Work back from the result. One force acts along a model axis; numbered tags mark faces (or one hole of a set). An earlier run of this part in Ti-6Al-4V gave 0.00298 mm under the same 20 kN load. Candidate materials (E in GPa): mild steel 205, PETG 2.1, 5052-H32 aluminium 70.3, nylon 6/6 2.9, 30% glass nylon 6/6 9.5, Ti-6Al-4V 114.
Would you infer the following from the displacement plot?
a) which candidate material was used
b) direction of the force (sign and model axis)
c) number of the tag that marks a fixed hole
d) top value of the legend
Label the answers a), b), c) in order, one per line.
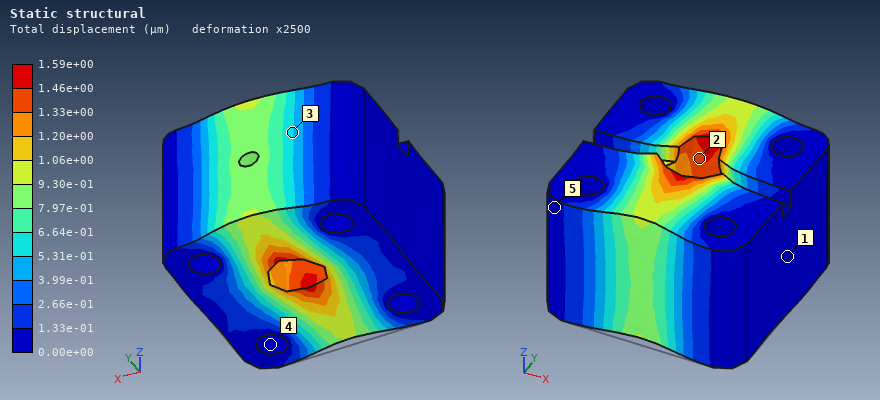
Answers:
a) mild steel
b) +Y
c) 4
d) 1.59e+00 µm
